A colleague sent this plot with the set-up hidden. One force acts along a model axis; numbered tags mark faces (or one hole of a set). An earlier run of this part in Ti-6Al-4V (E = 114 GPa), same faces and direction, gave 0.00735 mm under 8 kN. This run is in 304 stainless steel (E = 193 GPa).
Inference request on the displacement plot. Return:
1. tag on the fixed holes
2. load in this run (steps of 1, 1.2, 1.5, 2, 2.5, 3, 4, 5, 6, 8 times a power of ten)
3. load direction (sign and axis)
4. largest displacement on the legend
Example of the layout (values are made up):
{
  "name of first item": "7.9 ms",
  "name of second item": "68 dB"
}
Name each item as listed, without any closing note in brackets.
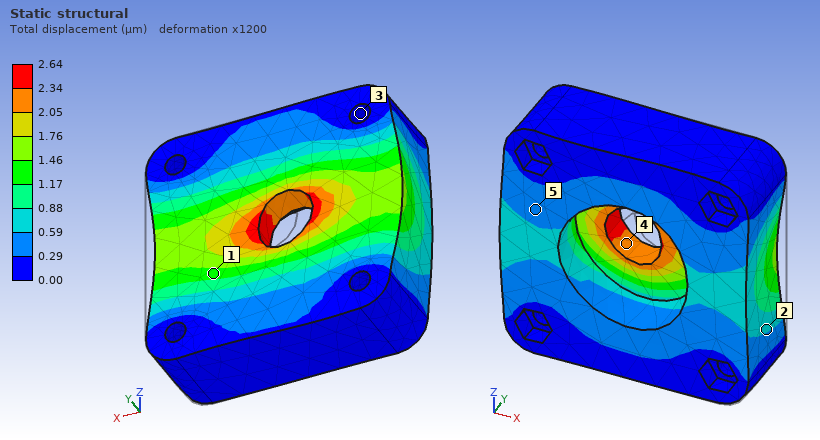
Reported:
{
  "tag on the fixed holes": "3",
  "load in this run": "5 kN",
  "load direction": "-X",
  "largest displacement on the legend": "2.64 µm"
}
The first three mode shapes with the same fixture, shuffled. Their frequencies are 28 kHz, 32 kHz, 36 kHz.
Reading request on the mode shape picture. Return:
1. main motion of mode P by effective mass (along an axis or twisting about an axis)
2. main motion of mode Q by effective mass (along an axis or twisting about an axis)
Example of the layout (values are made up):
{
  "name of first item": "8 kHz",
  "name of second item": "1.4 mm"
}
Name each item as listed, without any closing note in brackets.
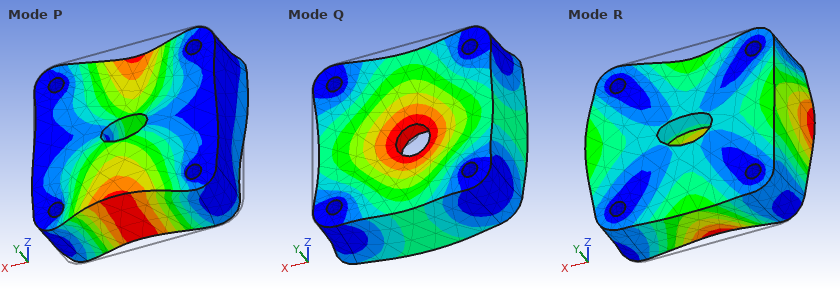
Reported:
{
  "main motion of mode P by effective mass": "twisting about X",
  "main motion of mode Q by effective mass": "along Y"
}
